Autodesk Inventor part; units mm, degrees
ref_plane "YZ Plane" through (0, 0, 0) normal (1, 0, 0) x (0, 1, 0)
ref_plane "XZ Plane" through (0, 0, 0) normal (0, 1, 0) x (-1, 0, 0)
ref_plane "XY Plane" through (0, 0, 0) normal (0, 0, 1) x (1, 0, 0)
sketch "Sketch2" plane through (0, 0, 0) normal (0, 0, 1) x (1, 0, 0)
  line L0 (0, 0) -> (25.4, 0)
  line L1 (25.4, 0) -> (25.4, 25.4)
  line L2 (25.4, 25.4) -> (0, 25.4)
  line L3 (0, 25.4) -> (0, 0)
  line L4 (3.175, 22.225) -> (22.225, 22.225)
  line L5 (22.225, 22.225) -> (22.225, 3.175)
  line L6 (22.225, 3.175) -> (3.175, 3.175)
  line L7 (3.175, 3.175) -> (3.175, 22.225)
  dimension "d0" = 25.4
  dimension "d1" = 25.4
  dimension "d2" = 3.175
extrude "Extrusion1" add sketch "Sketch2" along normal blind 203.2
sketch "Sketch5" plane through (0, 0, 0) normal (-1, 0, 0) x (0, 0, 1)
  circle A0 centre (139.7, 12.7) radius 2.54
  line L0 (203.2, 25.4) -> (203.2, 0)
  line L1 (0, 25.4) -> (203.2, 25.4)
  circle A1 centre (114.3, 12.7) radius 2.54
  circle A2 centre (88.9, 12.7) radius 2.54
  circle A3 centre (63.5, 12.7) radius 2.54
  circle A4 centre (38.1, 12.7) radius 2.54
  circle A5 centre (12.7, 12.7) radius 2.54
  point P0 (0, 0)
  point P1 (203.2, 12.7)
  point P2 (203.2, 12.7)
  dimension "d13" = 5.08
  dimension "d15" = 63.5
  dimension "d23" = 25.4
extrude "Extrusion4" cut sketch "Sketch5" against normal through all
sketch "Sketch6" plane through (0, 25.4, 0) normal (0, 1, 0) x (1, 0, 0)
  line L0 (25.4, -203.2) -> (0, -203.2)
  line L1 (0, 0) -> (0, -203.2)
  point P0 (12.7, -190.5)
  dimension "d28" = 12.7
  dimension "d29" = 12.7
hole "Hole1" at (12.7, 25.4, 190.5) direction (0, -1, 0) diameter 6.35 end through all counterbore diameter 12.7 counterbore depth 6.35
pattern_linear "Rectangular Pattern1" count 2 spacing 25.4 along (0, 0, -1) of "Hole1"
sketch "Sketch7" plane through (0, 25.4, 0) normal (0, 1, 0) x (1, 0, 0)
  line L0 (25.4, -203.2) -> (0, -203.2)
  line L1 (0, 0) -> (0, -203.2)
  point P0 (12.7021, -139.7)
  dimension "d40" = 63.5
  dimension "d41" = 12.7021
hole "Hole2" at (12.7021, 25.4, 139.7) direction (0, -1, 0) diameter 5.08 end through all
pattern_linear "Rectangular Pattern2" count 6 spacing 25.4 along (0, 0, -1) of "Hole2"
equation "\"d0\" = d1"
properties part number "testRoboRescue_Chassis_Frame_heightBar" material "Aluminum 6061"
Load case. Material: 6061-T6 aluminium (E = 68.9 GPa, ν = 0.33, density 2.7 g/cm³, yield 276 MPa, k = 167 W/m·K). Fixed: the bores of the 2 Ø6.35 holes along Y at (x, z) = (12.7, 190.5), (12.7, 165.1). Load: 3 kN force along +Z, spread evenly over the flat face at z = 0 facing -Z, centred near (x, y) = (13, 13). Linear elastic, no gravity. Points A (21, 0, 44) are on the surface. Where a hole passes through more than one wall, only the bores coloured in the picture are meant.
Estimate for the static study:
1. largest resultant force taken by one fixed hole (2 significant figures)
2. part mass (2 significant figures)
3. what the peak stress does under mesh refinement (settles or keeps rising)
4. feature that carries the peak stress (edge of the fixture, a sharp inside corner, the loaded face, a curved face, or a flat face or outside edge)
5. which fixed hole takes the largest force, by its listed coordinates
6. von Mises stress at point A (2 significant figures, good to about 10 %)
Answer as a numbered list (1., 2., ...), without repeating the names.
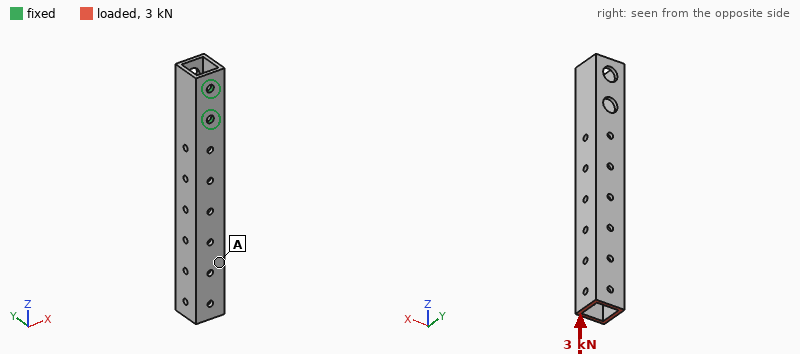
1. 2.2 kN
2. 150 g
3. keeps rising
4. edge of the fixture
5. (12.7, 165.1)
6. 12 MPa
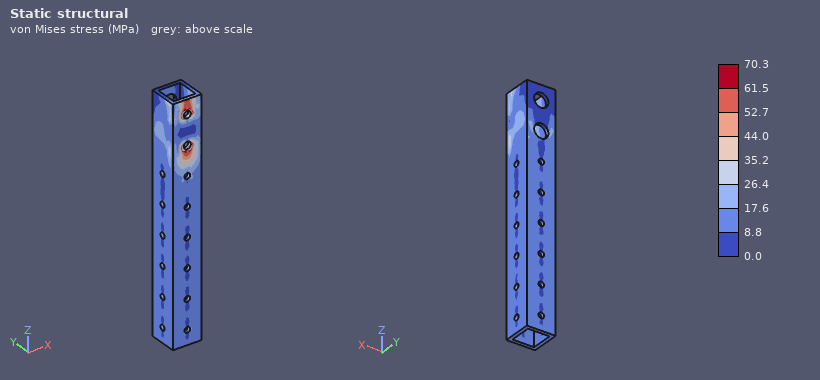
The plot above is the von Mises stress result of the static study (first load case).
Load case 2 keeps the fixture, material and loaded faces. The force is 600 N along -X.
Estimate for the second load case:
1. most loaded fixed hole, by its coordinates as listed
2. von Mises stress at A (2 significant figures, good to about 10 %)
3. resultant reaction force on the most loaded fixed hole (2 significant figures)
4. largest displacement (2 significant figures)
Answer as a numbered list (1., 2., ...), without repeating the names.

1. (12.7, 165.1)
2. 11 MPa
3. 3.4 kN
4. 1.1 mm
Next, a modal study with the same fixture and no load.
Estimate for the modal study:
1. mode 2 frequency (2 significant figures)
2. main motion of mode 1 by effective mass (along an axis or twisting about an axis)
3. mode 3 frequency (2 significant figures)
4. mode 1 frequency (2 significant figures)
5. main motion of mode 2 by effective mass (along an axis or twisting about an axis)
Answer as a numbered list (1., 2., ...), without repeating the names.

1. 630 Hz
2. along Y
3. 1700 Hz
4. 500 Hz
5. along X
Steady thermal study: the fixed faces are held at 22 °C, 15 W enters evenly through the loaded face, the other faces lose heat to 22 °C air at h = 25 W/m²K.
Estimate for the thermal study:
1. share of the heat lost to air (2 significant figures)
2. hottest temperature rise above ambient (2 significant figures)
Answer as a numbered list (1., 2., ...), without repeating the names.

1. 69 %
2. 32 K
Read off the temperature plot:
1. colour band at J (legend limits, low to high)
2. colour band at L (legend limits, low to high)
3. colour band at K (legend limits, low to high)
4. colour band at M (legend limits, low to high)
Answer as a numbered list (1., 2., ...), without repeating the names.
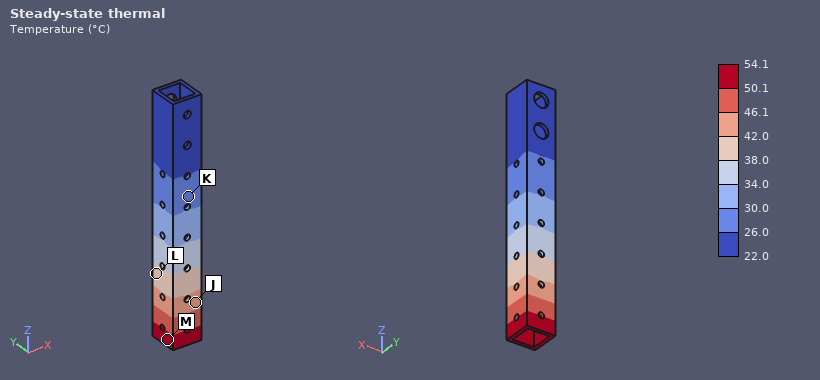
1. 42.0 to 46.1 °C
2. 38.0 to 42.0 °C
3. 26.0 to 30.0 °C
4. 50.1 to 54.1 °C
